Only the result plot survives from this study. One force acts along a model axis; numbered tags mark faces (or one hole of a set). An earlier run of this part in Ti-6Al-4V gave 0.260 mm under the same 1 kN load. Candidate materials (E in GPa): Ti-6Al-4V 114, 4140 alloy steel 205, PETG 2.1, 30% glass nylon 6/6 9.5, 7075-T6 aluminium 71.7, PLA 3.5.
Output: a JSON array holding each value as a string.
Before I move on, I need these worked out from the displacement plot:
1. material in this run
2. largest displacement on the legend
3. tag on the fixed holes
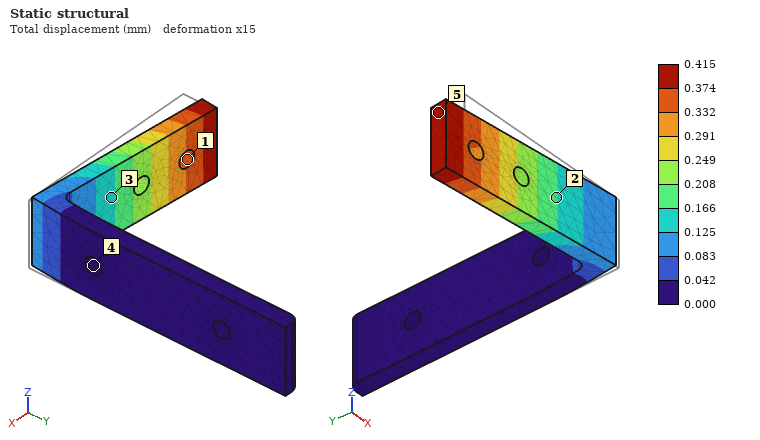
["7075-T6 aluminium", "0.415 mm", "4"]
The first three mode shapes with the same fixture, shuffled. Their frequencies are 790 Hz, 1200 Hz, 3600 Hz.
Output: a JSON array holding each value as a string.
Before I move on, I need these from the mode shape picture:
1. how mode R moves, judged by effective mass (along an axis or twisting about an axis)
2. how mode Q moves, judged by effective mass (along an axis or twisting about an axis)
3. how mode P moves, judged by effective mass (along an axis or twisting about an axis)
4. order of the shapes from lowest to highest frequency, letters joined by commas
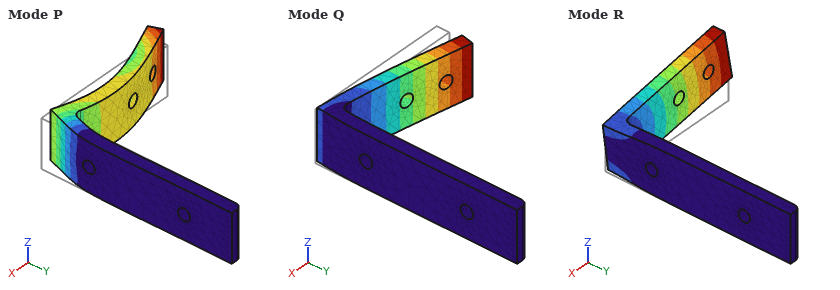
["along Z", "along Y", "along X", "Q, R, P"]
